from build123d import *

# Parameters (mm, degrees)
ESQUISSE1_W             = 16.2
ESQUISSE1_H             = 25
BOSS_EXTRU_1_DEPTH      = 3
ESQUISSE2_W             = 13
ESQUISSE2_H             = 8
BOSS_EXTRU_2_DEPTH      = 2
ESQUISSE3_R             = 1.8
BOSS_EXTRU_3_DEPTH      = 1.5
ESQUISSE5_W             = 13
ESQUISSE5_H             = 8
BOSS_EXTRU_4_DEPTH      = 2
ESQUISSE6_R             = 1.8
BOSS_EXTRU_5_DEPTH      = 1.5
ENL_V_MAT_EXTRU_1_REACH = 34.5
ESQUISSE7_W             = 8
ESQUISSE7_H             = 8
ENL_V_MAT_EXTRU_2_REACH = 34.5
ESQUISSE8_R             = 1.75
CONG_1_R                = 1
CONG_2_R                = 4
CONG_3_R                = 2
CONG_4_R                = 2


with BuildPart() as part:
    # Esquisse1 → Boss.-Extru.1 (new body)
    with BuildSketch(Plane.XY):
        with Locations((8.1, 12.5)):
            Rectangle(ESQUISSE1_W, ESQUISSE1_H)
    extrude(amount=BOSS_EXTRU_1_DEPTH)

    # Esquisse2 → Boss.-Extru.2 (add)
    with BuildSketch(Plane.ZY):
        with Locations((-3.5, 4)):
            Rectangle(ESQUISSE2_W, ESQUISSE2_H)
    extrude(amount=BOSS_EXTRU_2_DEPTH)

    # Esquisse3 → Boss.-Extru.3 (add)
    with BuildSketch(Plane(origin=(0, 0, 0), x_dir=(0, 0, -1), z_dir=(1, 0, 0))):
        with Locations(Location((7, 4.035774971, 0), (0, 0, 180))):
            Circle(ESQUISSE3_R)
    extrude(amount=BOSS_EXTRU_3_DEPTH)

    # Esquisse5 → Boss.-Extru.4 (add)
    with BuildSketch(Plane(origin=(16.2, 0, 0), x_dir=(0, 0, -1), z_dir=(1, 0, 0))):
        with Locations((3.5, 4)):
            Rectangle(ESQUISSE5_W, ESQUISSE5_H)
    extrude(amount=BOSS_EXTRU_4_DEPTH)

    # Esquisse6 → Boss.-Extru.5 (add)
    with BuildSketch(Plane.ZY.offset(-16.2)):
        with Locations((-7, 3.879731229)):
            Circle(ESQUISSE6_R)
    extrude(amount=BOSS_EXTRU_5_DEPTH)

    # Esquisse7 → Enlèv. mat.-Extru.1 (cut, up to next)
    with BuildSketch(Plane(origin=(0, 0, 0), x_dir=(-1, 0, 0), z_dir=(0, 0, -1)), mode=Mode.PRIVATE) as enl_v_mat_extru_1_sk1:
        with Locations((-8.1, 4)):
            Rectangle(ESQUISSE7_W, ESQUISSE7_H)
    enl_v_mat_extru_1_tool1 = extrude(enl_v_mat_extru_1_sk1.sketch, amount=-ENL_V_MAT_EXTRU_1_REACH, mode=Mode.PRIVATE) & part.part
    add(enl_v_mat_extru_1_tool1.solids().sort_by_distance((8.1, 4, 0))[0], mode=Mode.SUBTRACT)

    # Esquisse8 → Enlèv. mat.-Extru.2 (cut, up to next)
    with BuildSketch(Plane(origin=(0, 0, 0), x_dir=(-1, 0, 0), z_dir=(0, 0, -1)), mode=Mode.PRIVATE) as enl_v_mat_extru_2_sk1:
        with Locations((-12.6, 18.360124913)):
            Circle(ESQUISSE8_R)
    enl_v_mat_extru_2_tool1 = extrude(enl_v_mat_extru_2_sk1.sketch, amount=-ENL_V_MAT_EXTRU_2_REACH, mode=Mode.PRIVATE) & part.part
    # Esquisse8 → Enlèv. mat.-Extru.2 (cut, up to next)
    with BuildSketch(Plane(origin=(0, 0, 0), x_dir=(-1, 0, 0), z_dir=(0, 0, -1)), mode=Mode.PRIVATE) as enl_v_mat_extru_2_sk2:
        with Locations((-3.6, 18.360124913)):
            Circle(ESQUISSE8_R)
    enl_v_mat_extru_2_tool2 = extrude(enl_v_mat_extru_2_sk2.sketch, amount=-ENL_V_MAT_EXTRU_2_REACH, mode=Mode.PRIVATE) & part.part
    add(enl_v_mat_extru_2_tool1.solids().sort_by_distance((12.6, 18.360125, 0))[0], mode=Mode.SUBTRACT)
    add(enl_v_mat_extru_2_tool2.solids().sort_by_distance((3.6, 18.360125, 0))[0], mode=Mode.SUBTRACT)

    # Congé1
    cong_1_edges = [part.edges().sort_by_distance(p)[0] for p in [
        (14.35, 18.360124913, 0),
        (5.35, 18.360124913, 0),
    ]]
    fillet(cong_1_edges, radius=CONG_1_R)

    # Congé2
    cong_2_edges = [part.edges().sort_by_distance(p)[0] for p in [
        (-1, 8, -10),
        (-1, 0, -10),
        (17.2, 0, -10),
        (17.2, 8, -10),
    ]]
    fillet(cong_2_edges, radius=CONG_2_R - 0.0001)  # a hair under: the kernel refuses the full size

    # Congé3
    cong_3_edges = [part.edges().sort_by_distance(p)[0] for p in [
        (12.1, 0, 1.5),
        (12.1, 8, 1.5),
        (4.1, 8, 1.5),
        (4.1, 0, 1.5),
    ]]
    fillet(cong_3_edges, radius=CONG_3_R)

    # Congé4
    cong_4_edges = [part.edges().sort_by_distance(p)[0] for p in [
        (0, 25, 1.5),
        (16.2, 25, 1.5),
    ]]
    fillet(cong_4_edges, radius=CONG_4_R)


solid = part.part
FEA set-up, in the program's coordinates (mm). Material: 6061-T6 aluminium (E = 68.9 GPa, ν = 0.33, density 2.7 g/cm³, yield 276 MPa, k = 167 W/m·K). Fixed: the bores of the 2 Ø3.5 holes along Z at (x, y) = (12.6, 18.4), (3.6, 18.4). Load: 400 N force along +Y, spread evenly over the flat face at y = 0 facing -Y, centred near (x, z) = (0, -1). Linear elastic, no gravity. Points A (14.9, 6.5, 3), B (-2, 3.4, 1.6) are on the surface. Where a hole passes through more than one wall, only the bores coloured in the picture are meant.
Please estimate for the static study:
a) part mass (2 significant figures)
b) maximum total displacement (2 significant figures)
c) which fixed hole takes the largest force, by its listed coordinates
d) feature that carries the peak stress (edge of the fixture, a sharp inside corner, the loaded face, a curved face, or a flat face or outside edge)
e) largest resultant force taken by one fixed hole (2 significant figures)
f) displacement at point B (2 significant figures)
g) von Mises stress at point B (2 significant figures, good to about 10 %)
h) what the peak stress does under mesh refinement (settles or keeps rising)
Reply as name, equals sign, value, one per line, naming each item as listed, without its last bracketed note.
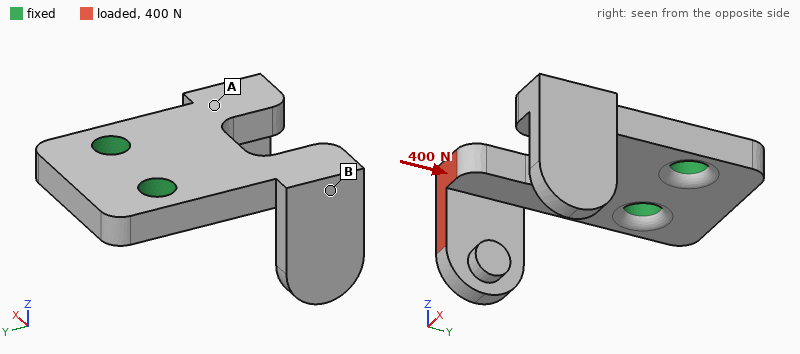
part mass = 3.7 g
maximum total displacement = 0.17 mm
which fixed hole takes the largest force, by its listed coordinates = (3.6, 18.4)
feature that carries the peak stress = a sharp inside corner
largest resultant force taken by one fixed hole = 520 N
displacement at point B = 0.082 mm
von Mises stress at point B = 34 MPa
what the peak stress does under mesh refinement = keeps rising
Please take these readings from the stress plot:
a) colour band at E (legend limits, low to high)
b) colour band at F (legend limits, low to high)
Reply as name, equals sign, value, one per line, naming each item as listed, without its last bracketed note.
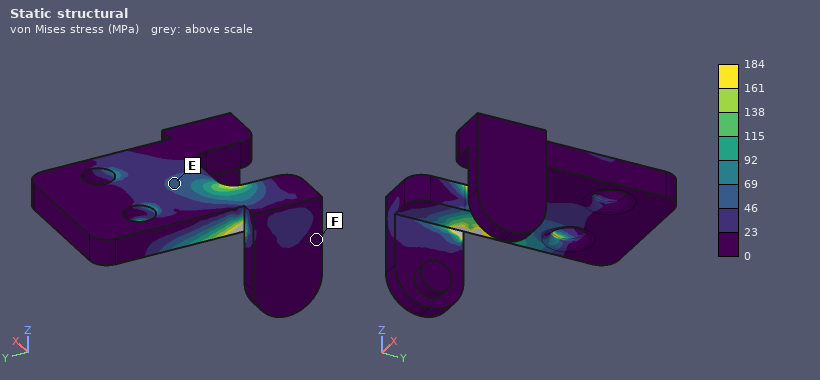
colour band at E = 46 to 69 MPa
colour band at F = 0 to 23 MPa
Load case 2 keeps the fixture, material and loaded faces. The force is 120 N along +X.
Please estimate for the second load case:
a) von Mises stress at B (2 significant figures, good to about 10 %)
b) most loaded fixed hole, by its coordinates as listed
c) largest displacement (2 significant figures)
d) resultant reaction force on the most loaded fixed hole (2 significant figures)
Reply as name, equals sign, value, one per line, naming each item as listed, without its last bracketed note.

von Mises stress at B = 27 MPa
most loaded fixed hole, by its coordinates as listed = (12.6, 18.4)
largest displacement = 72 µm
resultant reaction force on the most loaded fixed hole = 230 N
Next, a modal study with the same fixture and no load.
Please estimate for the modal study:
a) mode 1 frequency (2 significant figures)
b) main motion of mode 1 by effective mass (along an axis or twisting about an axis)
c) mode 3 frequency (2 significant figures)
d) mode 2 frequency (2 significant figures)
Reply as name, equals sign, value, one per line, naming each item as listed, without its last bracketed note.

mode 1 frequency = 5000 Hz
main motion of mode 1 by effective mass = along Z
mode 3 frequency = 8100 Hz
mode 2 frequency = 5700 Hz
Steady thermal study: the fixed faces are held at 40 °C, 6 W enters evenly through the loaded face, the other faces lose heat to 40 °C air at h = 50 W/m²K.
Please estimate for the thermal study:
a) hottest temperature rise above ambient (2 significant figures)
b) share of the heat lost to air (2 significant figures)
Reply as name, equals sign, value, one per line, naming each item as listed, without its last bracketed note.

hottest temperature rise above ambient = 29 K
share of the heat lost to air = 8.3 %
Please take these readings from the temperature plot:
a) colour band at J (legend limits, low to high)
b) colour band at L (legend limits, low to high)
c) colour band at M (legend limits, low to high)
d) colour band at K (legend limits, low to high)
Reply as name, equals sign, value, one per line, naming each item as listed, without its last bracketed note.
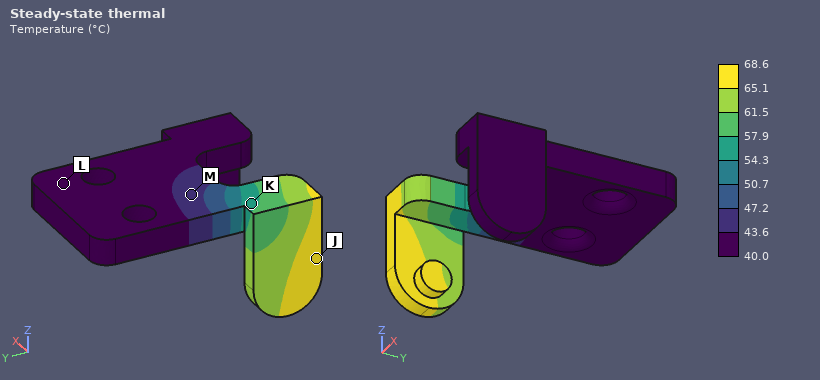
colour band at J = 65.1 to 68.6 °C
colour band at L = 40.0 to 43.6 °C
colour band at M = 43.6 to 47.2 °C
colour band at K = 54.3 to 57.9 °C
